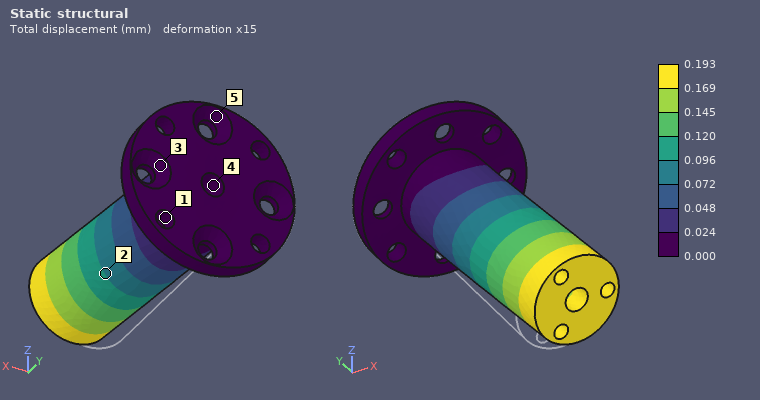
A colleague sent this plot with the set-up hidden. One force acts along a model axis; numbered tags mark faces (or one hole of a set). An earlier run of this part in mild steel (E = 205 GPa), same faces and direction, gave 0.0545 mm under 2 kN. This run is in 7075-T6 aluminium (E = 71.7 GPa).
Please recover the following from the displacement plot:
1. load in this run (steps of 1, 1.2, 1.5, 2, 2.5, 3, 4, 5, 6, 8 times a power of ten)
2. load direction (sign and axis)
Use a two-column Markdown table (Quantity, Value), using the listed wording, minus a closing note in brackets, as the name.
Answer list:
| Quantity | Value |
|---|---|
| load in this run | 2.5 kN |
| load direction | +X |
